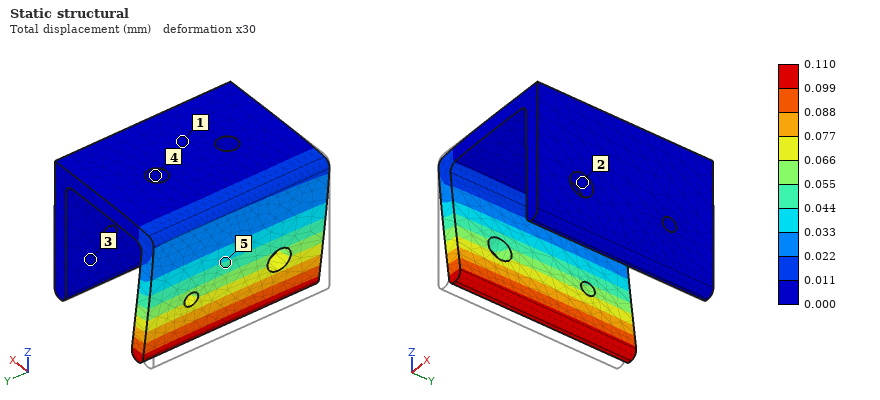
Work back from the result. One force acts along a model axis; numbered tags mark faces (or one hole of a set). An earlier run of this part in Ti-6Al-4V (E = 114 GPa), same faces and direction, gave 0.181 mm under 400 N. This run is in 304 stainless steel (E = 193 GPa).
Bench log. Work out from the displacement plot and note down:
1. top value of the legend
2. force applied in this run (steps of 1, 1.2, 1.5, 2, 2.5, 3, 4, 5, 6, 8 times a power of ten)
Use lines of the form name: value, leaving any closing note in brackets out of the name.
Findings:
top value of the legend: 0.110 mm
force applied in this run: 400 N
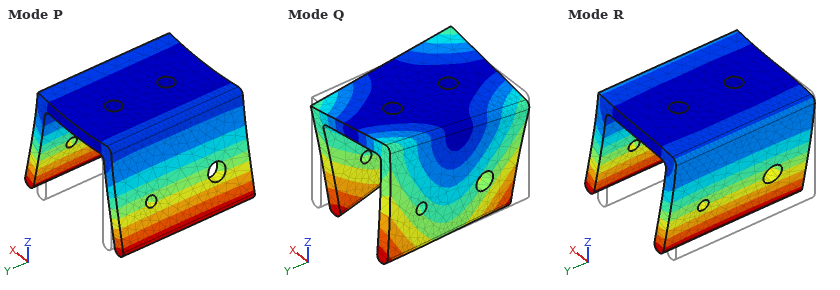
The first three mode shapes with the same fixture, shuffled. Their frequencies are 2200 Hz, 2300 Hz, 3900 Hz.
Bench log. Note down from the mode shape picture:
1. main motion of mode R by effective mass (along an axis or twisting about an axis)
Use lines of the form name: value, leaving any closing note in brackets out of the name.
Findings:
main motion of mode R by effective mass: along X
